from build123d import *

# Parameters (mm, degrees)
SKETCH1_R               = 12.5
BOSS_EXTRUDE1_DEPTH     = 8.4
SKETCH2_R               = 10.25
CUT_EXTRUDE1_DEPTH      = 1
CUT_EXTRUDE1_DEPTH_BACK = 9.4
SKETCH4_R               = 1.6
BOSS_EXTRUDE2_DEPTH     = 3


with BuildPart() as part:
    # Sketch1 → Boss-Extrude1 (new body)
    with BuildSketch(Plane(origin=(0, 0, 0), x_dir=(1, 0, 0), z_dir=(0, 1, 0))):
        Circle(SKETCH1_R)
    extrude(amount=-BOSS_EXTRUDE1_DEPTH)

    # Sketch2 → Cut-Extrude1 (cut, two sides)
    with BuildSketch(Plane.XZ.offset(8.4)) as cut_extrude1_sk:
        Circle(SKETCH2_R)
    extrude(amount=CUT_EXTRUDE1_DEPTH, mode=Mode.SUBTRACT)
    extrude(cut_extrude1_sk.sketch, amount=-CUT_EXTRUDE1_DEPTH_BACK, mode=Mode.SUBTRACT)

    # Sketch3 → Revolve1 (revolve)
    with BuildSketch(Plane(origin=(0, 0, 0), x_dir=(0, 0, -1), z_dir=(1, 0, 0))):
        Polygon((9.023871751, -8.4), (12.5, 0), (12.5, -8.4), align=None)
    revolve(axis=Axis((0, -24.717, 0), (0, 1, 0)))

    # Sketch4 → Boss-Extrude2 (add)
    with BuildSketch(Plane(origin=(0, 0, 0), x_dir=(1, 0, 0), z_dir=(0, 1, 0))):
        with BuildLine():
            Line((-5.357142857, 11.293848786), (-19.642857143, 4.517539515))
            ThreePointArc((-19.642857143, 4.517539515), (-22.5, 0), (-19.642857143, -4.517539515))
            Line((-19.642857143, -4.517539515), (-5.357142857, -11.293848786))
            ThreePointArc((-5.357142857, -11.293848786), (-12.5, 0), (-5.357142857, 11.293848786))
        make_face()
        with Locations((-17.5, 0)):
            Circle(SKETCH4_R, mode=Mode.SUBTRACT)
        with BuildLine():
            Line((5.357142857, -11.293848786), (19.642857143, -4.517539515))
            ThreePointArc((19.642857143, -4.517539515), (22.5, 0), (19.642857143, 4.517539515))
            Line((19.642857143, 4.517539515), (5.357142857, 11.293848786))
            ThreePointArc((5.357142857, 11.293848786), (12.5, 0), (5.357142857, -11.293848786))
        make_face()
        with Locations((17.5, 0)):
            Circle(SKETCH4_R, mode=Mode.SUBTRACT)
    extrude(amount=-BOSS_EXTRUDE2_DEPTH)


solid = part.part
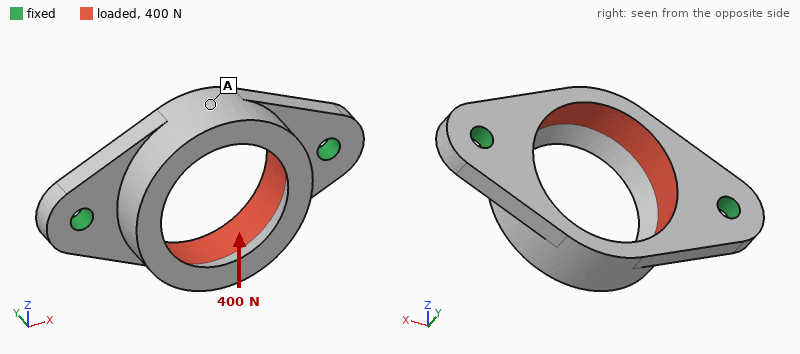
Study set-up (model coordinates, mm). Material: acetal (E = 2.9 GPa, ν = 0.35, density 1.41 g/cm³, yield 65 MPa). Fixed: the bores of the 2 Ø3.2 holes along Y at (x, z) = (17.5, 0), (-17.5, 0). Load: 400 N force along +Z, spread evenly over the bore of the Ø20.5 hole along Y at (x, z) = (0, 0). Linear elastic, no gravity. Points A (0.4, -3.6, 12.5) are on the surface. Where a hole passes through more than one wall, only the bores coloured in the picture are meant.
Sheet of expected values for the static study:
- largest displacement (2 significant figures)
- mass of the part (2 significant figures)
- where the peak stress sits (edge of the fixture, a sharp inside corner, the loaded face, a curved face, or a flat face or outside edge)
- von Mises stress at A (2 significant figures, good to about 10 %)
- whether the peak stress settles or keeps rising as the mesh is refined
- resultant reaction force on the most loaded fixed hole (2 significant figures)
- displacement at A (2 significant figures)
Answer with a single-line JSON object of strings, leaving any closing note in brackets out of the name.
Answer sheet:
{"largest displacement": "0.21 mm", "mass of the part": "3.1 g", "where the peak stress sits": "edge of the fixture", "von Mises stress at A": "3.8 MPa", "whether the peak stress settles or keeps rising as the mesh is refined": "keeps rising", "resultant reaction force on the most loaded fixed hole": "200 N", "displacement at A": "0.19 mm"}
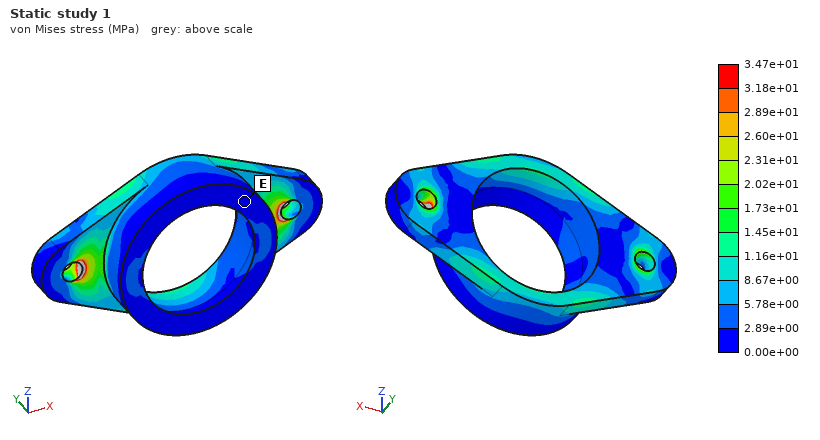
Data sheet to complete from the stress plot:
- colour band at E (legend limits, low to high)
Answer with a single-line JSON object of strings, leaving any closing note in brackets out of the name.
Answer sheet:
{"colour band at E": "0.00e+00 to 2.89e+00 MPa"}
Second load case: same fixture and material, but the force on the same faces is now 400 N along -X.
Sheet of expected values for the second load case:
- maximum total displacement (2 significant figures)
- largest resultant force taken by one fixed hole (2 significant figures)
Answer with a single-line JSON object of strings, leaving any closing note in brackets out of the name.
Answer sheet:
{"maximum total displacement": "70 µm", "largest resultant force taken by one fixed hole": "200 N"}
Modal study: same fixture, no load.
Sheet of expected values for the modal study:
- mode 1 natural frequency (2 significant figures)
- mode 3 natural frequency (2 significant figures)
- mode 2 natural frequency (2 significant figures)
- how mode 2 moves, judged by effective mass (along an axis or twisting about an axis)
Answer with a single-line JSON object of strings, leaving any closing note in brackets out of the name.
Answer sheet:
{"mode 1 natural frequency": "2400 Hz", "mode 3 natural frequency": "5700 Hz", "mode 2 natural frequency": "3600 Hz", "how mode 2 moves, judged by effective mass": "along Y"}
